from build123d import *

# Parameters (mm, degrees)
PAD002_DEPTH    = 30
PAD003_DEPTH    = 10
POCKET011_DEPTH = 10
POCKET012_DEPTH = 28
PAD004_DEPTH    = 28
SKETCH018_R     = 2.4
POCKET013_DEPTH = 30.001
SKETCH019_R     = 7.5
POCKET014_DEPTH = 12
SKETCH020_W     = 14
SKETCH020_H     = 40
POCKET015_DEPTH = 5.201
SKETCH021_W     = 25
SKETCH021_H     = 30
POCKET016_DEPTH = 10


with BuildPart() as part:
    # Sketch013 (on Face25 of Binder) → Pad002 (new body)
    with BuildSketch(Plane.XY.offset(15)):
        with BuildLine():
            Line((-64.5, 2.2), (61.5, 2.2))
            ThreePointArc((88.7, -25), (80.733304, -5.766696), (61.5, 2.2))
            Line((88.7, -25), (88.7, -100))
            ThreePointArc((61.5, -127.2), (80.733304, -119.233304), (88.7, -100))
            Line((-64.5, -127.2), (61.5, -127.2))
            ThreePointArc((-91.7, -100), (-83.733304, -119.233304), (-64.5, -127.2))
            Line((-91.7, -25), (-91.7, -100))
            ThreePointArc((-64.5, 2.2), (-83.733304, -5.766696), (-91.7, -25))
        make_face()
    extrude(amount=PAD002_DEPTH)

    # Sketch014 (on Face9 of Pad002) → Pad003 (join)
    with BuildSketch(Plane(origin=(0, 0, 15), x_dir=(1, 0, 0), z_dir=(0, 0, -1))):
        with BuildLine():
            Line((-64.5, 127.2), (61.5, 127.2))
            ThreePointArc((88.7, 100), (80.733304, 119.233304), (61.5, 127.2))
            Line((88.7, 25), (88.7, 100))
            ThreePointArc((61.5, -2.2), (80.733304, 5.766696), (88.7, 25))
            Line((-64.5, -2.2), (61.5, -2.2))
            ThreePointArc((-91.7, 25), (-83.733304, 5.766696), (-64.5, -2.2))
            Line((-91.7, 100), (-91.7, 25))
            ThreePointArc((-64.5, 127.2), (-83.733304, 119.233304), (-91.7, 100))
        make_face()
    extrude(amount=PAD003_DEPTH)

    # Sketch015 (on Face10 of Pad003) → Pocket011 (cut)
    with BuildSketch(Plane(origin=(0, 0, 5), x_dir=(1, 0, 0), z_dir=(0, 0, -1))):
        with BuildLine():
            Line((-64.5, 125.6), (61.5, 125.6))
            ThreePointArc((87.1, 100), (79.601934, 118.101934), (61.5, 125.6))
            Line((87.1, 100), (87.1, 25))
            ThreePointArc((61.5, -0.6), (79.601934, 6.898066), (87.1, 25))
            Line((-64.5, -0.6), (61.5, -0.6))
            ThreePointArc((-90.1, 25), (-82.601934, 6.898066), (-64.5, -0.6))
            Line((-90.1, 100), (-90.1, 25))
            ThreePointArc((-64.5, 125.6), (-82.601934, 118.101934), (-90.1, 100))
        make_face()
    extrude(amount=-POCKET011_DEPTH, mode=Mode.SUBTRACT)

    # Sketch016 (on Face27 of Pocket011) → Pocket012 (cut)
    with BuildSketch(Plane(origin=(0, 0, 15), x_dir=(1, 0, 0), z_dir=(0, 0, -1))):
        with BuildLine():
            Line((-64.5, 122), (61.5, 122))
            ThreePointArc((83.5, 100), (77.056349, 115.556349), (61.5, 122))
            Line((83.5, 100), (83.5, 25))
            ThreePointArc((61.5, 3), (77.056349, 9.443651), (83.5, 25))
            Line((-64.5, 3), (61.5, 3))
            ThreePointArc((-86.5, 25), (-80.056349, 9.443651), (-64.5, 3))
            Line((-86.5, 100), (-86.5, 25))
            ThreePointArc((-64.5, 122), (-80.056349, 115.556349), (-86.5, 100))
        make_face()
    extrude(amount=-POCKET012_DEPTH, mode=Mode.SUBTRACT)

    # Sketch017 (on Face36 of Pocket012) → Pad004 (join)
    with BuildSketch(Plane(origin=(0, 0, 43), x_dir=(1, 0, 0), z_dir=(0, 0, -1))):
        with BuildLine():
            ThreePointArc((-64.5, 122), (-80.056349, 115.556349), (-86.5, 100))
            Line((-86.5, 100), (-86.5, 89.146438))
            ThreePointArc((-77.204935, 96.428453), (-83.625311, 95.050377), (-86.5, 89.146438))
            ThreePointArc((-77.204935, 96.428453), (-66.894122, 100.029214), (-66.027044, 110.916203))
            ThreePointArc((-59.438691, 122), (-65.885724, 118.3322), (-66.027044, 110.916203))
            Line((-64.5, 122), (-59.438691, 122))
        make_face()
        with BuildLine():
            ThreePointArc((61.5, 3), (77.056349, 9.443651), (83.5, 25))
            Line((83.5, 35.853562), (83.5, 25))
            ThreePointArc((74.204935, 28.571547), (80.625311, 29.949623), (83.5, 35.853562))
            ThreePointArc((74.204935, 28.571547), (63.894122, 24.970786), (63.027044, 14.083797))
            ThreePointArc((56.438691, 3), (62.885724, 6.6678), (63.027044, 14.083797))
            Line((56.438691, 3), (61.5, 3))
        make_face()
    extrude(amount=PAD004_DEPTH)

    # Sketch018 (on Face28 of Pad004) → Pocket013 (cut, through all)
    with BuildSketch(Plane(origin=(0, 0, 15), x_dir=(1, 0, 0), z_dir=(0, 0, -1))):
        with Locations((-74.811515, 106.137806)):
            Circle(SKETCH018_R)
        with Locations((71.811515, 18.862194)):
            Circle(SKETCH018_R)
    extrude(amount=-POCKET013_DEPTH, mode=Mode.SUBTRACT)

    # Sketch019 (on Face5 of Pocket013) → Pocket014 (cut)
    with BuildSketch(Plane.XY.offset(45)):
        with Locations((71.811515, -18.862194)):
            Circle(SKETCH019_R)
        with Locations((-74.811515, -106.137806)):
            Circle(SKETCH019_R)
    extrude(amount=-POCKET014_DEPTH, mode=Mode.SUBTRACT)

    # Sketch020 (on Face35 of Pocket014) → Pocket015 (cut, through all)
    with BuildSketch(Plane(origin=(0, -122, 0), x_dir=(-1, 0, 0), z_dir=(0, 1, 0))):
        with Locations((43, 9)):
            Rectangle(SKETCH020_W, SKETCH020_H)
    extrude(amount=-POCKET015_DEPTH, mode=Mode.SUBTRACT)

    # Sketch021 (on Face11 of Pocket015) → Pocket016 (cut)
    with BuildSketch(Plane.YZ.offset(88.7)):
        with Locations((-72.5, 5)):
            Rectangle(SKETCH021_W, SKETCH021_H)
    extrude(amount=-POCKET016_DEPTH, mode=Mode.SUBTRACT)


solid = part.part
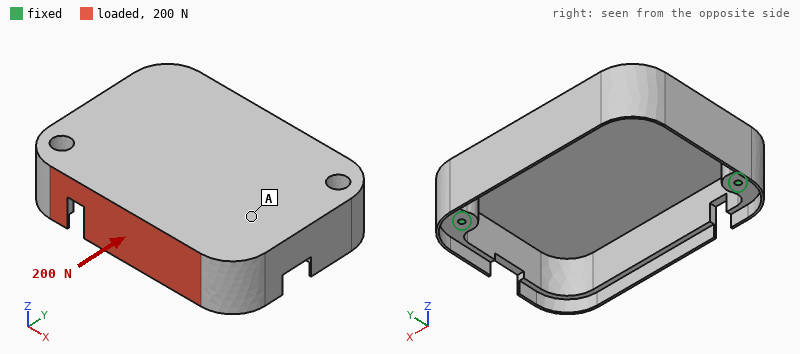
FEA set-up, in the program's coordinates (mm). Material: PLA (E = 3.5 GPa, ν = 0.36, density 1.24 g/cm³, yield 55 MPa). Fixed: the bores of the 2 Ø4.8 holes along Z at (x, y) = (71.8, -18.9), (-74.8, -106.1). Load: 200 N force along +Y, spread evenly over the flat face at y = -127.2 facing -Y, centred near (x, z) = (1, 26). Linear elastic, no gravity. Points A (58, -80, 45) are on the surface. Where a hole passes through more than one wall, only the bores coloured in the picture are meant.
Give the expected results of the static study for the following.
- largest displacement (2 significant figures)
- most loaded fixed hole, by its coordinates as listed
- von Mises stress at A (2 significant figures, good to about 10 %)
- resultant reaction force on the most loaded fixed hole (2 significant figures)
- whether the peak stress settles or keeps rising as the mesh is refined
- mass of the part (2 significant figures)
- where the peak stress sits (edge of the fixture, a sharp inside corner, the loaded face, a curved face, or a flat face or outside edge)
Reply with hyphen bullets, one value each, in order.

- 1.6 mm
- (71.8, -18.9)
- 1.3 MPa
- 120 N
- keeps rising
- 190 g
- a sharp inside corner
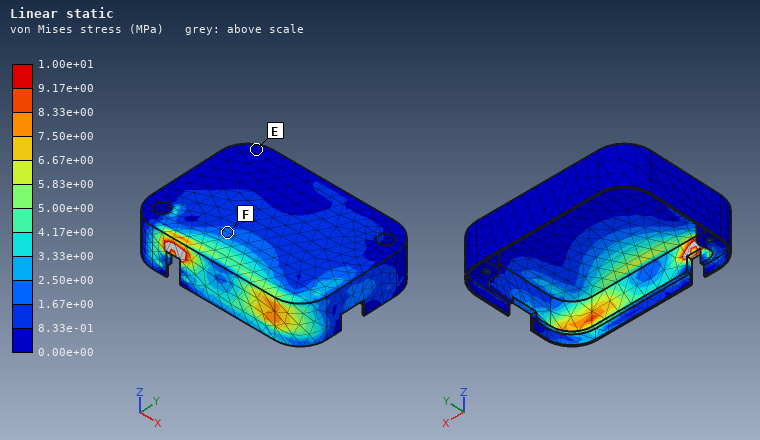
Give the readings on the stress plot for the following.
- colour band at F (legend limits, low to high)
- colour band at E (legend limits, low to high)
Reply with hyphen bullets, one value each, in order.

- 1.67e+00 to 2.50e+00 MPa
- 0.00e+00 to 8.33e-01 MPa
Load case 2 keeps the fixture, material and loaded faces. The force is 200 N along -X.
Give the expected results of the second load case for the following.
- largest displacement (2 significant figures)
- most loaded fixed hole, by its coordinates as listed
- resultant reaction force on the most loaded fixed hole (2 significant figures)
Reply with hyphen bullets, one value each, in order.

- 0.20 mm
- (-74.8, -106.1)
- 190 N
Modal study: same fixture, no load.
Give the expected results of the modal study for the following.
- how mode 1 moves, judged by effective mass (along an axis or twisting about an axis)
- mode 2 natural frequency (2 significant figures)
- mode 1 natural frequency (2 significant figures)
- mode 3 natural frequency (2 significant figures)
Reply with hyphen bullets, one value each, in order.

- along Z
- 400 Hz
- 300 Hz
- 510 Hz
